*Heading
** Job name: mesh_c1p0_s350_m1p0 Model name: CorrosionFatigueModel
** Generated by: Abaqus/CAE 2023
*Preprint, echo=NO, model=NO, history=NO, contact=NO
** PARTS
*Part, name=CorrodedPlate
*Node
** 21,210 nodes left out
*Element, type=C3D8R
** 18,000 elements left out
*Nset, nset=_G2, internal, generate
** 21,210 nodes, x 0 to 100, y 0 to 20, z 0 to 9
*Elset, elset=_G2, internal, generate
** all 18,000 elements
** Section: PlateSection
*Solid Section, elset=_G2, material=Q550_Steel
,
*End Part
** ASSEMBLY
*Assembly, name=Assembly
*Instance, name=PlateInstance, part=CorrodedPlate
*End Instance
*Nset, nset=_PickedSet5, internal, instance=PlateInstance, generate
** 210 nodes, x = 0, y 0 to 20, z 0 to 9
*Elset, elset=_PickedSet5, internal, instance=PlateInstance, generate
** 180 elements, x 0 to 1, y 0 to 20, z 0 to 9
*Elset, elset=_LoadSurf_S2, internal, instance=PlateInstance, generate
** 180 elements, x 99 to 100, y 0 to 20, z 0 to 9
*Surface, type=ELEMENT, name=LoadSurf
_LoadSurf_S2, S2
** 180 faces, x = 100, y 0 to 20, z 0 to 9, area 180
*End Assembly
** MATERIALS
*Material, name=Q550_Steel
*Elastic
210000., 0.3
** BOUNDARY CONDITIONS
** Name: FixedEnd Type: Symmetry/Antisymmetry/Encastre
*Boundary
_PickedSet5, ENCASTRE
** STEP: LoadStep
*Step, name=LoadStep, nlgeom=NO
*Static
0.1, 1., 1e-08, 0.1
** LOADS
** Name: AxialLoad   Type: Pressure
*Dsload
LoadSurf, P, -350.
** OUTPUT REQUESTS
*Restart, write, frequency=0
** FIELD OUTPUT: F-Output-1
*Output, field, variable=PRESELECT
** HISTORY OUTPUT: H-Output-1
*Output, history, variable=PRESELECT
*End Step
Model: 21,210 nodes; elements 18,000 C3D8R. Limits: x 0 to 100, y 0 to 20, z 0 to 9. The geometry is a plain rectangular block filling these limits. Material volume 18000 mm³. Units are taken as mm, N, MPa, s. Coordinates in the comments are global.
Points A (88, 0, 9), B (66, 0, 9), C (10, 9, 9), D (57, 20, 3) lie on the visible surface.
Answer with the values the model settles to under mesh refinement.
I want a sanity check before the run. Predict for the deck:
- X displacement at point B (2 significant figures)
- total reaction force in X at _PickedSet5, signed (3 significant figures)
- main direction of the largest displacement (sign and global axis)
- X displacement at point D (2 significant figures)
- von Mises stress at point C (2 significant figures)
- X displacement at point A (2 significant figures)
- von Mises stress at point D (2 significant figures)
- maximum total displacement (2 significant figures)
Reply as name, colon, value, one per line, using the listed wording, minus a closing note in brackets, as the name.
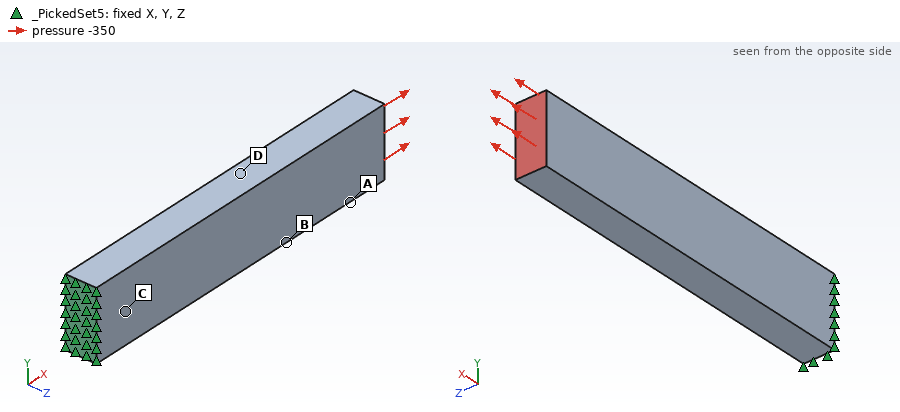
X displacement at point B: 0.11 mm
total reaction force in X at _PickedSet5, signed: -63000 N
main direction of the largest displacement: +X
X displacement at point D: 0.094 mm
von Mises stress at point C: 360 MPa
X displacement at point A: 0.15 mm
von Mises stress at point D: 350 MPa
maximum total displacement: 0.17 mm
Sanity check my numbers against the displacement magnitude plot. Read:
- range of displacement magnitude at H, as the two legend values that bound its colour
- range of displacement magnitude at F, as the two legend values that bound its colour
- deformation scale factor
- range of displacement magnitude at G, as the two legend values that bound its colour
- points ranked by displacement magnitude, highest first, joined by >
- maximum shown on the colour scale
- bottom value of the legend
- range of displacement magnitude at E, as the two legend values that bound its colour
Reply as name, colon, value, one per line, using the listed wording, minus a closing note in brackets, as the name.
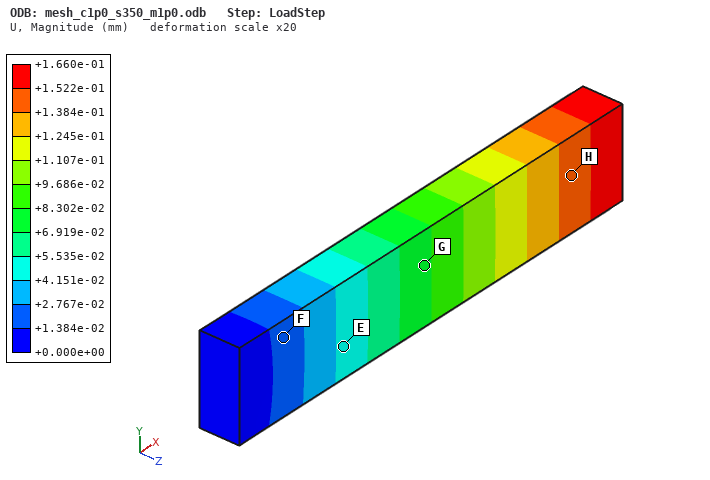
range of displacement magnitude at H, as the two legend values that bound its colour: +1.384e-01 to +1.522e-01 mm
range of displacement magnitude at F, as the two legend values that bound its colour: +1.384e-02 to +2.767e-02 mm
deformation scale factor: 20
range of displacement magnitude at G, as the two legend values that bound its colour: +6.919e-02 to +8.302e-02 mm
points ranked by displacement magnitude, highest first, joined by >: H > G > E > F
maximum shown on the colour scale: +1.660e-01 mm
bottom value of the legend: +0.000e+00 mm
range of displacement magnitude at E, as the two legend values that bound its colour: +4.151e-02 to +5.535e-02 mm
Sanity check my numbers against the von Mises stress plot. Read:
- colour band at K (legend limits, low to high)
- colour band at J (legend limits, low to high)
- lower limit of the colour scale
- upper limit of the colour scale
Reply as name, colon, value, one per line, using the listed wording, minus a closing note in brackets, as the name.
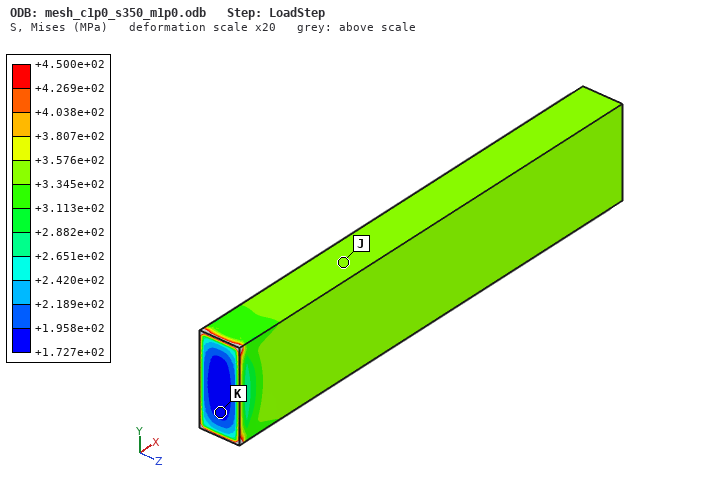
colour band at K: +1.727e+02 to +1.958e+02 MPa
colour band at J: +3.345e+02 to +3.576e+02 MPa
lower limit of the colour scale: +1.727e+02 MPa
upper limit of the colour scale: +4.500e+02 MPa
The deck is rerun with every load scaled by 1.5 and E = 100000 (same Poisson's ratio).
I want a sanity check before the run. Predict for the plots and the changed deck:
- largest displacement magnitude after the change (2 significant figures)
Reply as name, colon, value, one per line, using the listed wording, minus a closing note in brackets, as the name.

largest displacement magnitude after the change: 0.52 mm
